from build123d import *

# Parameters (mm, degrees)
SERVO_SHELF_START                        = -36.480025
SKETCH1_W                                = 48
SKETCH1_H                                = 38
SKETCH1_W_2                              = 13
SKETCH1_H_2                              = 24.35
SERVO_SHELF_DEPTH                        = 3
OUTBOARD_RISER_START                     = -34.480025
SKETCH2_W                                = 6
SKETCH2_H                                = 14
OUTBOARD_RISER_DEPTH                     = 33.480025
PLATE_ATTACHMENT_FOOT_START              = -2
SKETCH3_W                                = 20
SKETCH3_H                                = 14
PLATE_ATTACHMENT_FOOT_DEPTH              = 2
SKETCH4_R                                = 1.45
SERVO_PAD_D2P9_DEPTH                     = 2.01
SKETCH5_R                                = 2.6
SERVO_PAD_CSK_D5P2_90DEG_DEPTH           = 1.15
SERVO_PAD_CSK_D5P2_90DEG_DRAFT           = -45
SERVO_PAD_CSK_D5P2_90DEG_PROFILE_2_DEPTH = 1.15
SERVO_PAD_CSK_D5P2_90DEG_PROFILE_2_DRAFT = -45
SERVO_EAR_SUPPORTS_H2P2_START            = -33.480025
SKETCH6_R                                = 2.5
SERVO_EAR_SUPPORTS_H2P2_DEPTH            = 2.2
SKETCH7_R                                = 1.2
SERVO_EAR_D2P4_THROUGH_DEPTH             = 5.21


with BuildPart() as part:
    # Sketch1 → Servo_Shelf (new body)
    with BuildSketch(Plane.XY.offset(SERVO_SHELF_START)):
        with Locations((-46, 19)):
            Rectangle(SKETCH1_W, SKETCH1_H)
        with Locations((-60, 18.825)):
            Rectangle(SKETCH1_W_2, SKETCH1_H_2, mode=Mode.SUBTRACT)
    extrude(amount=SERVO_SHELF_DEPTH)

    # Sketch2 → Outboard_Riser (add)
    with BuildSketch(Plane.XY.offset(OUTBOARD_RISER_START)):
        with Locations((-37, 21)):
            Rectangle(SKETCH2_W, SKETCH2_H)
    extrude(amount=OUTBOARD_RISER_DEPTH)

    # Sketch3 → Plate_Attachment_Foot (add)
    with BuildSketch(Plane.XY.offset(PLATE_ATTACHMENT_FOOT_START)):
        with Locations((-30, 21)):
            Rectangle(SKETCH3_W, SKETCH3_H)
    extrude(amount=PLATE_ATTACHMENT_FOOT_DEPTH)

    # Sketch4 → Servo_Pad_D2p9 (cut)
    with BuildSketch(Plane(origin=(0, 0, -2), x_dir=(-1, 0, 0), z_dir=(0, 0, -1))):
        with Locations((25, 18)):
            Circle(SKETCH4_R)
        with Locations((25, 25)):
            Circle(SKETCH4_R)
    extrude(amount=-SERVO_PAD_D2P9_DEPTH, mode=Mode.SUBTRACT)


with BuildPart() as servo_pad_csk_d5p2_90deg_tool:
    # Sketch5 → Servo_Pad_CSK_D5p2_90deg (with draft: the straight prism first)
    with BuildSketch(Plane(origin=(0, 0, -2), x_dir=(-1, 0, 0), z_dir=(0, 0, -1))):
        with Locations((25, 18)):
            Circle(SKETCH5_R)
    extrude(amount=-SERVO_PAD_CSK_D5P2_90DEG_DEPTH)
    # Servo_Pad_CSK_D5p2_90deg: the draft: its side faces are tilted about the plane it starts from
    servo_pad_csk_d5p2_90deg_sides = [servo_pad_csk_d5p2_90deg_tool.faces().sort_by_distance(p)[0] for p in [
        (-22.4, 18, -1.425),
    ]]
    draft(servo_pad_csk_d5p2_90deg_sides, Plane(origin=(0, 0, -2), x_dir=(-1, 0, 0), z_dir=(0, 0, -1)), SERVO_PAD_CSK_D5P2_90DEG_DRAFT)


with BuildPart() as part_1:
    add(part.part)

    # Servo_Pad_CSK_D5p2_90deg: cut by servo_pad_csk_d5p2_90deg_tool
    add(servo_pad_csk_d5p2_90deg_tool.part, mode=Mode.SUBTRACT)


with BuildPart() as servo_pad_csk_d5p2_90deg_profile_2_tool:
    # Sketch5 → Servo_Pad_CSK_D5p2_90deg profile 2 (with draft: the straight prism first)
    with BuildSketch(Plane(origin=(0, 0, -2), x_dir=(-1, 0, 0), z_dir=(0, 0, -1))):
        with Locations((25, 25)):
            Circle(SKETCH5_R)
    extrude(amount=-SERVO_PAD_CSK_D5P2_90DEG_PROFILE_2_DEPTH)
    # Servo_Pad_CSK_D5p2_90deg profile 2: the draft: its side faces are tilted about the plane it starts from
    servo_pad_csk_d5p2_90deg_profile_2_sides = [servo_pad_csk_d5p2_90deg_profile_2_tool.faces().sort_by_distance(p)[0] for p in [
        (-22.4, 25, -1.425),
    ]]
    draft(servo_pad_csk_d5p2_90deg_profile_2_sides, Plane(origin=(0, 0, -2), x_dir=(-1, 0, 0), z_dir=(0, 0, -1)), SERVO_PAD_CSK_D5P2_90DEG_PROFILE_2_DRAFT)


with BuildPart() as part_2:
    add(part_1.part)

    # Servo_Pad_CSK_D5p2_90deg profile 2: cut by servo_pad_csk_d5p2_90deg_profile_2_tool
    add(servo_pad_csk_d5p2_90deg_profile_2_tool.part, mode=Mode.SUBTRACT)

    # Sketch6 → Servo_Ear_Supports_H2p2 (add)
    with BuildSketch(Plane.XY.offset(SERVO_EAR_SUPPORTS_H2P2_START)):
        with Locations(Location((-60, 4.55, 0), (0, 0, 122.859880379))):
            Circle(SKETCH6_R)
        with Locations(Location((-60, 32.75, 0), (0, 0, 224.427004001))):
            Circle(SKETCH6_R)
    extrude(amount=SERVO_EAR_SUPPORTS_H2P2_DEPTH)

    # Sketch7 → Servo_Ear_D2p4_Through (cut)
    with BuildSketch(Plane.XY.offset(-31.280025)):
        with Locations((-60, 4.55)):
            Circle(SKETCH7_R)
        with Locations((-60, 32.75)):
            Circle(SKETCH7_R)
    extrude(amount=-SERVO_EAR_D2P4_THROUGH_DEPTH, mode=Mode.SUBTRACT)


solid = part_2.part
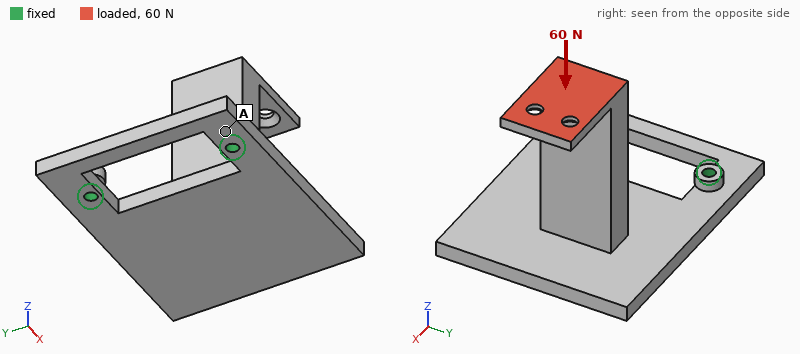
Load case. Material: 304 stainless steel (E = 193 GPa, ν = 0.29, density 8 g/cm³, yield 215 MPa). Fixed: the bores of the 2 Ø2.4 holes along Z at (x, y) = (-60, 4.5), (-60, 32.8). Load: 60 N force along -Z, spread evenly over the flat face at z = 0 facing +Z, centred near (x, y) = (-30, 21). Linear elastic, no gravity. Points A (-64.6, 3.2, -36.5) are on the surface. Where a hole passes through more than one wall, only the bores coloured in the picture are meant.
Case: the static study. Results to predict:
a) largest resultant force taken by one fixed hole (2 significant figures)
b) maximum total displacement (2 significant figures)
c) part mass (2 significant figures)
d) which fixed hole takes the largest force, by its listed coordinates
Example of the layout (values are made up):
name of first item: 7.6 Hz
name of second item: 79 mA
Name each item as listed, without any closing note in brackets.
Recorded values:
largest resultant force taken by one fixed hole: 34 N
maximum total displacement: 0.16 mm
part mass: 62 g
which fixed hole takes the largest force, by its listed coordinates: (-60, 32.8)
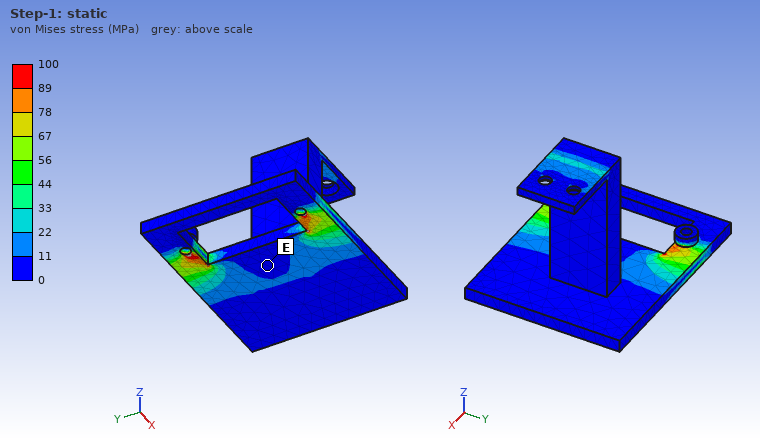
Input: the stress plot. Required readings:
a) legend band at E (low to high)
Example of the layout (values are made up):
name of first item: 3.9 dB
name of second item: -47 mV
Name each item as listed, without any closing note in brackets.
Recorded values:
legend band at E: 0 to 11 MPa
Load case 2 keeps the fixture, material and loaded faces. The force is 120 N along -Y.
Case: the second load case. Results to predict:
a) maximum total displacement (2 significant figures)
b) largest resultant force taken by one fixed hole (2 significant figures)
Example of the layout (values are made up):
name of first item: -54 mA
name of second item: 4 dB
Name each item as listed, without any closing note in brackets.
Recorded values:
maximum total displacement: 95 µm
largest resultant force taken by one fixed hole: 180 N
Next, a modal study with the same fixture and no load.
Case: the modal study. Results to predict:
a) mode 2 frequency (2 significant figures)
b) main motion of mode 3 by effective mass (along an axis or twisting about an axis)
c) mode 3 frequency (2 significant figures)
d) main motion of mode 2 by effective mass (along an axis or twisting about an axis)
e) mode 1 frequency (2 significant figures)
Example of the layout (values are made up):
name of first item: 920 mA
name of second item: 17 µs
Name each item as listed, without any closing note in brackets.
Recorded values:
mode 2 frequency: 1700 Hz
main motion of mode 3 by effective mass: along Z
mode 3 frequency: 2600 Hz
main motion of mode 2 by effective mass: along Y
mode 1 frequency: 620 Hz
